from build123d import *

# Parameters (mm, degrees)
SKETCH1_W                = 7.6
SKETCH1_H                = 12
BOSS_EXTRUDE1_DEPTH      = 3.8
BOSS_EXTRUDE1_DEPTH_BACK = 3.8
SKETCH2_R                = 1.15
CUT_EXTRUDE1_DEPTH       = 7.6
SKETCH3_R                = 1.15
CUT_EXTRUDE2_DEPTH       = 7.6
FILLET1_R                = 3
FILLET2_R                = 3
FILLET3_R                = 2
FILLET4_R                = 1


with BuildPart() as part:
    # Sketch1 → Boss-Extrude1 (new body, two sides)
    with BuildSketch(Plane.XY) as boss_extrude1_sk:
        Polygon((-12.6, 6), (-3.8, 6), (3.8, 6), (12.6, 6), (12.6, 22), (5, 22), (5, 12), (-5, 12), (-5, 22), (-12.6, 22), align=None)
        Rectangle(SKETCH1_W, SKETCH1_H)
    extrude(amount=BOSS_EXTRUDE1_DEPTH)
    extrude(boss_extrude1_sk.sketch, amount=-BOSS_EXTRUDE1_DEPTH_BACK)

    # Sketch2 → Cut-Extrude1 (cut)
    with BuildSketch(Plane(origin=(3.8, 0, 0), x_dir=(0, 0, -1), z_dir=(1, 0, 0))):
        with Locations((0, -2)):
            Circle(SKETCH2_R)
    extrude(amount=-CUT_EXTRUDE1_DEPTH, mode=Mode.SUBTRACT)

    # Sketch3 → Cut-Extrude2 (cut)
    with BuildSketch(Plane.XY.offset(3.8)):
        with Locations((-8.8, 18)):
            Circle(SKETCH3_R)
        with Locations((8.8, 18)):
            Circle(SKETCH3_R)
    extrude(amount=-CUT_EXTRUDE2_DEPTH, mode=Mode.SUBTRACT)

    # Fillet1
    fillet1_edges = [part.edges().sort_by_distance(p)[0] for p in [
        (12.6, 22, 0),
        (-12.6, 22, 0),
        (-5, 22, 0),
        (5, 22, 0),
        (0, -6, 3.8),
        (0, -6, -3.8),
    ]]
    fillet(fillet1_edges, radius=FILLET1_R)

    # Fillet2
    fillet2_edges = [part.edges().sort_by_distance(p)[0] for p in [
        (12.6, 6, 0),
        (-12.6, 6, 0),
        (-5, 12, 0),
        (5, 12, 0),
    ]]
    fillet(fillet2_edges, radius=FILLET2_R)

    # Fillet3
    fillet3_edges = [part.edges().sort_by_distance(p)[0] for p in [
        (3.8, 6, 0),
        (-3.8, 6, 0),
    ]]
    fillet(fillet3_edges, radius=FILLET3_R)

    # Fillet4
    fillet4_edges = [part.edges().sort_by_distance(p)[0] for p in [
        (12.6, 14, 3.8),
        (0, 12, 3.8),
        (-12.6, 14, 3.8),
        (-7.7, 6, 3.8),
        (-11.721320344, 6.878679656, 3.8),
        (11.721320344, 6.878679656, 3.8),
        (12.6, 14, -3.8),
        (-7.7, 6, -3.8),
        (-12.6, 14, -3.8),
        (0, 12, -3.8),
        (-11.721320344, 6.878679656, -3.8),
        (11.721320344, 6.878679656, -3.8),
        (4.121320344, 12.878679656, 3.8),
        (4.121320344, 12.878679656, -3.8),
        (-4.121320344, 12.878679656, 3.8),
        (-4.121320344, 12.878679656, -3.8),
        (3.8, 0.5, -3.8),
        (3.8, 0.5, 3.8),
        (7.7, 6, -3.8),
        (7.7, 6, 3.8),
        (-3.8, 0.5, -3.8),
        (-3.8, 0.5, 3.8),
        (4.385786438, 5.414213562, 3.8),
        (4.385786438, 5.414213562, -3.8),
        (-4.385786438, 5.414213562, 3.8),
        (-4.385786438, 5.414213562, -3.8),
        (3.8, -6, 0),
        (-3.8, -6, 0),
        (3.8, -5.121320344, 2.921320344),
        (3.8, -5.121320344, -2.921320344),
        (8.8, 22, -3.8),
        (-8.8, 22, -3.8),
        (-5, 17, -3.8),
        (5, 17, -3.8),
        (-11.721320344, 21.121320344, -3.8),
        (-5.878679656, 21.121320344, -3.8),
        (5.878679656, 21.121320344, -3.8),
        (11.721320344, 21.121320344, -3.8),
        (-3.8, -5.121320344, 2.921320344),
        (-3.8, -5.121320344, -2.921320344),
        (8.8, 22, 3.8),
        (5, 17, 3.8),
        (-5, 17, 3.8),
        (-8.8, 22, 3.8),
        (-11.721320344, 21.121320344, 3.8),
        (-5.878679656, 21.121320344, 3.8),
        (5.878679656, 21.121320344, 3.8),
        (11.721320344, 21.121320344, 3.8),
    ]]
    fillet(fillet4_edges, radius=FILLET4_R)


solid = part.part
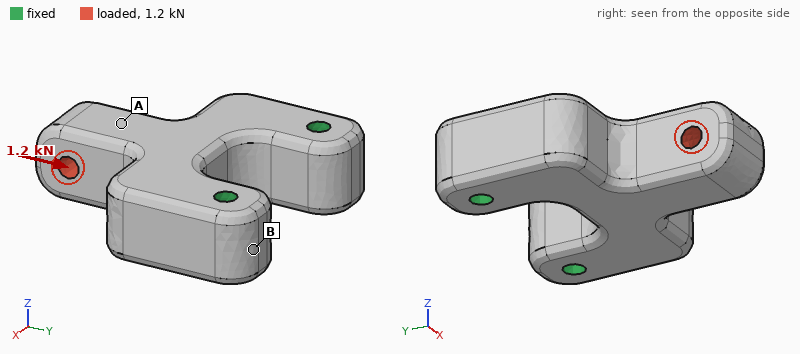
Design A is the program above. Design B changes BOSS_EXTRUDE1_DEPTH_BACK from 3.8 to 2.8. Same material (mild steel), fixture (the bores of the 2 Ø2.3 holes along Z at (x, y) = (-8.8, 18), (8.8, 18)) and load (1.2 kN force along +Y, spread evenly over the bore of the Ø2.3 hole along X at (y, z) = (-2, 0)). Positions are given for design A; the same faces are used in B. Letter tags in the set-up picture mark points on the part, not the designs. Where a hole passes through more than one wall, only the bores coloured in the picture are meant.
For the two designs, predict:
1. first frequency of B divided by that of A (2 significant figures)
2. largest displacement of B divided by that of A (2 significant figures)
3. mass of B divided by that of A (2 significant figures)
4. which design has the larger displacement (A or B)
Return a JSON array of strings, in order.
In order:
["0.90", "1.9", "0.86", "B"]
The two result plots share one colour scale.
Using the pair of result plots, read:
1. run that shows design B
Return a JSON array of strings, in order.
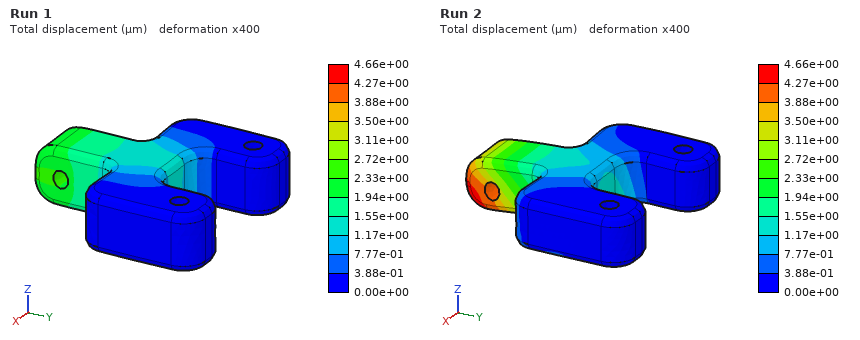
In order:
["Run 2"]
